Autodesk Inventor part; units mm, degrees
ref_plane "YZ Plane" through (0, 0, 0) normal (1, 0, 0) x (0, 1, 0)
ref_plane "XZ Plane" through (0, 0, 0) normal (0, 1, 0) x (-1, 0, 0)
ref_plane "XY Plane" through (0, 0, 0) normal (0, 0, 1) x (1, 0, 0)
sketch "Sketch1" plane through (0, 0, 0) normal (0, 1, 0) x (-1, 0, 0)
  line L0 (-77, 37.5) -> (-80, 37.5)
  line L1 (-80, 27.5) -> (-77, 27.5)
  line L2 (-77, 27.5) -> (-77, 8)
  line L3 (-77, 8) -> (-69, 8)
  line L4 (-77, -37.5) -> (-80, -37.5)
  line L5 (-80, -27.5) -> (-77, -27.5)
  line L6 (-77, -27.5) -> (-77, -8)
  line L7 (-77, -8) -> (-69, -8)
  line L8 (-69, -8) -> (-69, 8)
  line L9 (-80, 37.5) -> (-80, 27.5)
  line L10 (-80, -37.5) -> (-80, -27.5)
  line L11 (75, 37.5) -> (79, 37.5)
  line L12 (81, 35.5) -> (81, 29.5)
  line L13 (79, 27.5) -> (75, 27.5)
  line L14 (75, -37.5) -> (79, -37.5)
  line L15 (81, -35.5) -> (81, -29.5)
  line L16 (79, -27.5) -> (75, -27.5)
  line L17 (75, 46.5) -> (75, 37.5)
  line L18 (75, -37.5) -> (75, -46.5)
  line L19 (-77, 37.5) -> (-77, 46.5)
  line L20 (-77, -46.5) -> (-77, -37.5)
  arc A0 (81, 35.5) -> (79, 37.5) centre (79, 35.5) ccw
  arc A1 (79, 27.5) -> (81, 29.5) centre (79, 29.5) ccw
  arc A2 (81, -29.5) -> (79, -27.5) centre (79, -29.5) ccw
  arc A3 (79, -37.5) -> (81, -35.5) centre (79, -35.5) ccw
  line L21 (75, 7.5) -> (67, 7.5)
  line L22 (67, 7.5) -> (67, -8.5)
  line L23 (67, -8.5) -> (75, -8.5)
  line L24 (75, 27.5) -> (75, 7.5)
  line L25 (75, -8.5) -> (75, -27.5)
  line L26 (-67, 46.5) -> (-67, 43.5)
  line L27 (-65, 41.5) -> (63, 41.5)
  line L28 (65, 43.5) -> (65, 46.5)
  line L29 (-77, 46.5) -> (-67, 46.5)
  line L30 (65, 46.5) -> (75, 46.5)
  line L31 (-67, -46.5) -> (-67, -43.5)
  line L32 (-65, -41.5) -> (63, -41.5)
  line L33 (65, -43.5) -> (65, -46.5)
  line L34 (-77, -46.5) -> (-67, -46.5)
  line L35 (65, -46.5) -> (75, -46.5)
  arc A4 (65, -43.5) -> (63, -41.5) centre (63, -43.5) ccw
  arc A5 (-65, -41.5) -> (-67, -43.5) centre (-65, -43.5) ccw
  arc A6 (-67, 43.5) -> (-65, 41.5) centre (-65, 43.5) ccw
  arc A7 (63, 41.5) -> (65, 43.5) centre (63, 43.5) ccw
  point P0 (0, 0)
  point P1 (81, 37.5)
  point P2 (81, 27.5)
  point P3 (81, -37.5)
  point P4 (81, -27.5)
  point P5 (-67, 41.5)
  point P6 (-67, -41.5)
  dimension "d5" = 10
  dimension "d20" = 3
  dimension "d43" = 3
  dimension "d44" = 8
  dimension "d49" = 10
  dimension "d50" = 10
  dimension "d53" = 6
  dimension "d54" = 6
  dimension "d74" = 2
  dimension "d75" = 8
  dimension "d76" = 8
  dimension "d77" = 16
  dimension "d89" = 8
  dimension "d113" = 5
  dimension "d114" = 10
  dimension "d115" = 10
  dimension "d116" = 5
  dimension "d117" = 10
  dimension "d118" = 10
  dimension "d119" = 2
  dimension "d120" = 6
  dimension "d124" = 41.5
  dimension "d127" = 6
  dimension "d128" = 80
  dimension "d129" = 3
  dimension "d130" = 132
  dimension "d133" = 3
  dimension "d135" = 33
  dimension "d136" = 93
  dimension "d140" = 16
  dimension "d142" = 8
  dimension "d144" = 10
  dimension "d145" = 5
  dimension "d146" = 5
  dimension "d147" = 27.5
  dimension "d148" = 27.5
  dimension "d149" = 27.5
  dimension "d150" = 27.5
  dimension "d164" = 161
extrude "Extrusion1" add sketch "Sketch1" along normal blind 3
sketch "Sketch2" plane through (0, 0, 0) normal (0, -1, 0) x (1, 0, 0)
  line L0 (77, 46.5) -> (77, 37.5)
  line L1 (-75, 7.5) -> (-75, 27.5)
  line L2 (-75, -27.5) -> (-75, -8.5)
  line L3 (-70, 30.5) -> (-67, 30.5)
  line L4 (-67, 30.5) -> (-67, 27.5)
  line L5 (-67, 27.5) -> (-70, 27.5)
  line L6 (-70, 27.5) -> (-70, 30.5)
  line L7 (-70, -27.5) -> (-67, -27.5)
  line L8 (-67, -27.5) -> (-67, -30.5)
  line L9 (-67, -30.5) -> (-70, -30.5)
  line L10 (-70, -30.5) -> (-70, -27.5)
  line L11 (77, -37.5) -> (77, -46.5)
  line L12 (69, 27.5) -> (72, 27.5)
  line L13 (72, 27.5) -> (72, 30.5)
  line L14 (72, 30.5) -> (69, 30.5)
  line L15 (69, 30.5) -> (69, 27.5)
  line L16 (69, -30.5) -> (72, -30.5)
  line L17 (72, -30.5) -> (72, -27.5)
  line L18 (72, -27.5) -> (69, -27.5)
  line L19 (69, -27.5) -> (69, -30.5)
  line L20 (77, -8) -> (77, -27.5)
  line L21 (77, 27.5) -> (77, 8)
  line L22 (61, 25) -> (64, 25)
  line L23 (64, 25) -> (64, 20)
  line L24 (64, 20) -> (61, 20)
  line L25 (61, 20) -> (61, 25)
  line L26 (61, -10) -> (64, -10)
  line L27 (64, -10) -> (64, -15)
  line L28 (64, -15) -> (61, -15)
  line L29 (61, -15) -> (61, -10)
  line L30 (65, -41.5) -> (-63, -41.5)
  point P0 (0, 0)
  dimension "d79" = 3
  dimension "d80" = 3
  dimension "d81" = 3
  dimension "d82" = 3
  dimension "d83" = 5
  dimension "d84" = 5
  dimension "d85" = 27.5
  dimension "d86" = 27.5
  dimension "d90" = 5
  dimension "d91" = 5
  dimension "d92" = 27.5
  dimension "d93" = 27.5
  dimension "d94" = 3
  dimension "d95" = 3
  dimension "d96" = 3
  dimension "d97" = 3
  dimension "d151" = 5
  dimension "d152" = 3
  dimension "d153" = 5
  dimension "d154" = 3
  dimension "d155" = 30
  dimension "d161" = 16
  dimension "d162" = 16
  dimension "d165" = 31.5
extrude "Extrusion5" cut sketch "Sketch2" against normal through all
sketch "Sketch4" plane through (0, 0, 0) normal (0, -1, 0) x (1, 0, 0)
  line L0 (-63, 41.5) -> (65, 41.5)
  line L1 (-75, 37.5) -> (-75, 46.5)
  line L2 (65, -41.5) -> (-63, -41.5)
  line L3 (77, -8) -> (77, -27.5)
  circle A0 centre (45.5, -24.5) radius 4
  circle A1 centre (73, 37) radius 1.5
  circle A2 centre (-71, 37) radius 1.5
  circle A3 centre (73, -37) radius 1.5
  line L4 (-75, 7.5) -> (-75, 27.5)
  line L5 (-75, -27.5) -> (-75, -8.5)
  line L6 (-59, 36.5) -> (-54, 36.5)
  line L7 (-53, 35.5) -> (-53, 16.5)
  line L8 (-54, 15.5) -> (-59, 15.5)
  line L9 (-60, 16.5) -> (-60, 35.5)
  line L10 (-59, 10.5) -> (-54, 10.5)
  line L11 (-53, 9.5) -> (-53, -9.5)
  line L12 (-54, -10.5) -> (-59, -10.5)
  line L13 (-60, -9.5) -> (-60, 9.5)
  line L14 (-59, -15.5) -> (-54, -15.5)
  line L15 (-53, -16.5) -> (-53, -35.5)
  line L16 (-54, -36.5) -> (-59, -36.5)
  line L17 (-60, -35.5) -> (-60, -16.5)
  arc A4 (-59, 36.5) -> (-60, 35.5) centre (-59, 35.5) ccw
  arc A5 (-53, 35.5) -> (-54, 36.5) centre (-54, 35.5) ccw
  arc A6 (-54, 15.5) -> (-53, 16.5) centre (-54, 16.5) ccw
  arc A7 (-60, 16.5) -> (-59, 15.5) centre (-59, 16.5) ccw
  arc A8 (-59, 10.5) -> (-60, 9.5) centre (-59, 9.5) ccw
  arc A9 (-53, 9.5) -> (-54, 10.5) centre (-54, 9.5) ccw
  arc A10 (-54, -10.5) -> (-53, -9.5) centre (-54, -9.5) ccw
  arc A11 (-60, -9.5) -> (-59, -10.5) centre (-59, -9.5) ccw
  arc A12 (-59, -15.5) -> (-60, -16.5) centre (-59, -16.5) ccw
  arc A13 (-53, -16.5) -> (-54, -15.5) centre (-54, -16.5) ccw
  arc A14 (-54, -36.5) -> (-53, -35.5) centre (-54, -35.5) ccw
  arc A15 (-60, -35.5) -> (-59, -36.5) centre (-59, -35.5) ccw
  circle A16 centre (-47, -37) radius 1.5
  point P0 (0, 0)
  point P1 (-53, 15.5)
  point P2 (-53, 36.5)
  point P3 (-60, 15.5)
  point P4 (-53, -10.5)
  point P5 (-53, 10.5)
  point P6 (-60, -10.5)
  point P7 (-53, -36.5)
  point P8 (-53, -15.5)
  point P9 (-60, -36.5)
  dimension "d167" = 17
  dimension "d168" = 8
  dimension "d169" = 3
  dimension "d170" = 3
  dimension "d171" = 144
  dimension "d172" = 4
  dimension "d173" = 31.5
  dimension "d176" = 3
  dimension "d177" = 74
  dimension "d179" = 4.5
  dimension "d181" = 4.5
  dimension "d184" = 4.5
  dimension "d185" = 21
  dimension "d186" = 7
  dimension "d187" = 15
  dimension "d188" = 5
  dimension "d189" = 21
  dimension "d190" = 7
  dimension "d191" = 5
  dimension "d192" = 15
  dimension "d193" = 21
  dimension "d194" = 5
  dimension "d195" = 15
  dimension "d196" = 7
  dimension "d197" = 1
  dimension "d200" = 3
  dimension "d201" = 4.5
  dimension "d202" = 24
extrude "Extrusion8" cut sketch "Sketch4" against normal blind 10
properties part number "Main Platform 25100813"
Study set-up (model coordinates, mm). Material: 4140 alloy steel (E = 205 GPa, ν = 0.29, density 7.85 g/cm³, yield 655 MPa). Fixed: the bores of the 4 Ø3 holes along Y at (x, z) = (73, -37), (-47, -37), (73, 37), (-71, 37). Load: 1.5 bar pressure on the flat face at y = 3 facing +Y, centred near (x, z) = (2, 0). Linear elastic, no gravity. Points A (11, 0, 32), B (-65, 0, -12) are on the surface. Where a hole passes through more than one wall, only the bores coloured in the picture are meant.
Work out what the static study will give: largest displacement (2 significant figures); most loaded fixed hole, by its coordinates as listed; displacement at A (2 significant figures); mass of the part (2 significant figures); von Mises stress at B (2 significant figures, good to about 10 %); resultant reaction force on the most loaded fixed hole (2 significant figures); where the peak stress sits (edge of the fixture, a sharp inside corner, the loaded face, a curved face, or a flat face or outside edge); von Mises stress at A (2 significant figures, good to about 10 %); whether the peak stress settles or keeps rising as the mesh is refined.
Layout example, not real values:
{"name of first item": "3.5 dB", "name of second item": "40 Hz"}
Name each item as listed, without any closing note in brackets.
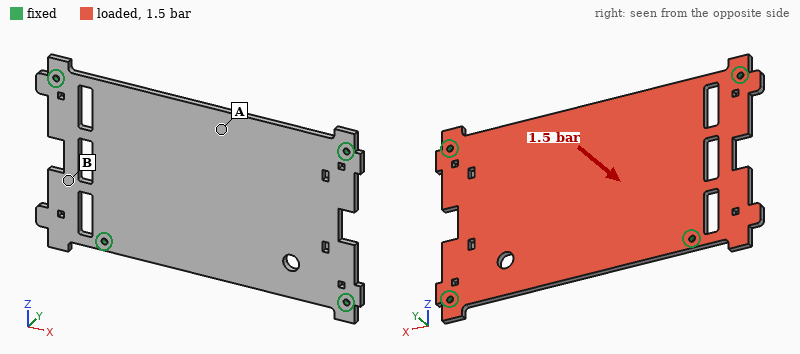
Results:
{"largest displacement": "0.52 mm", "most loaded fixed hole, by its coordinates as listed": "(-47, -37)", "displacement at A": "0.48 mm", "mass of the part": "290 g", "von Mises stress at B": "50 MPa", "resultant reaction force on the most loaded fixed hole": "600 N", "where the peak stress sits": "edge of the fixture", "von Mises stress at A": "98 MPa", "whether the peak stress settles or keeps rising as the mesh is refined": "keeps rising"}
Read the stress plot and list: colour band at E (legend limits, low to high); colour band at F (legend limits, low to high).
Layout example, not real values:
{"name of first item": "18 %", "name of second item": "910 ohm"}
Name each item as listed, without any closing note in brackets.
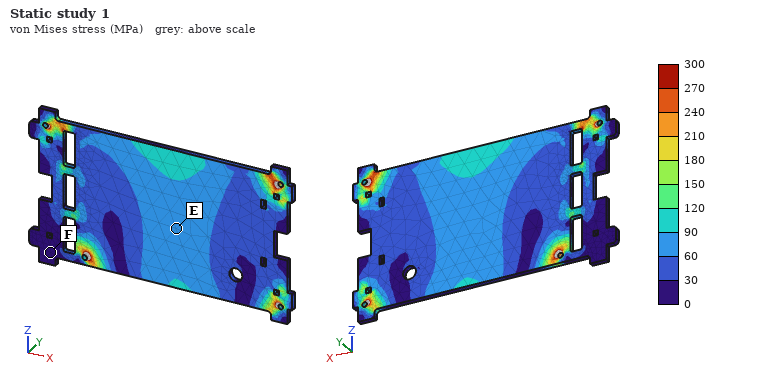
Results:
{"colour band at E": "60 to 90 MPa", "colour band at F": "0 to 30 MPa"}
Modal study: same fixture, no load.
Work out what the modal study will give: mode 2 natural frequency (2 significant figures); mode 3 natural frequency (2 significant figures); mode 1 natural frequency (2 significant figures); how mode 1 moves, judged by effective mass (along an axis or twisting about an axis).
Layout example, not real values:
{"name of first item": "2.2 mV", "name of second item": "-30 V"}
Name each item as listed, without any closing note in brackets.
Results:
{"mode 2 natural frequency": "1300 Hz", "mode 3 natural frequency": "1800 Hz", "mode 1 natural frequency": "690 Hz", "how mode 1 moves, judged by effective mass": "along Y"}
